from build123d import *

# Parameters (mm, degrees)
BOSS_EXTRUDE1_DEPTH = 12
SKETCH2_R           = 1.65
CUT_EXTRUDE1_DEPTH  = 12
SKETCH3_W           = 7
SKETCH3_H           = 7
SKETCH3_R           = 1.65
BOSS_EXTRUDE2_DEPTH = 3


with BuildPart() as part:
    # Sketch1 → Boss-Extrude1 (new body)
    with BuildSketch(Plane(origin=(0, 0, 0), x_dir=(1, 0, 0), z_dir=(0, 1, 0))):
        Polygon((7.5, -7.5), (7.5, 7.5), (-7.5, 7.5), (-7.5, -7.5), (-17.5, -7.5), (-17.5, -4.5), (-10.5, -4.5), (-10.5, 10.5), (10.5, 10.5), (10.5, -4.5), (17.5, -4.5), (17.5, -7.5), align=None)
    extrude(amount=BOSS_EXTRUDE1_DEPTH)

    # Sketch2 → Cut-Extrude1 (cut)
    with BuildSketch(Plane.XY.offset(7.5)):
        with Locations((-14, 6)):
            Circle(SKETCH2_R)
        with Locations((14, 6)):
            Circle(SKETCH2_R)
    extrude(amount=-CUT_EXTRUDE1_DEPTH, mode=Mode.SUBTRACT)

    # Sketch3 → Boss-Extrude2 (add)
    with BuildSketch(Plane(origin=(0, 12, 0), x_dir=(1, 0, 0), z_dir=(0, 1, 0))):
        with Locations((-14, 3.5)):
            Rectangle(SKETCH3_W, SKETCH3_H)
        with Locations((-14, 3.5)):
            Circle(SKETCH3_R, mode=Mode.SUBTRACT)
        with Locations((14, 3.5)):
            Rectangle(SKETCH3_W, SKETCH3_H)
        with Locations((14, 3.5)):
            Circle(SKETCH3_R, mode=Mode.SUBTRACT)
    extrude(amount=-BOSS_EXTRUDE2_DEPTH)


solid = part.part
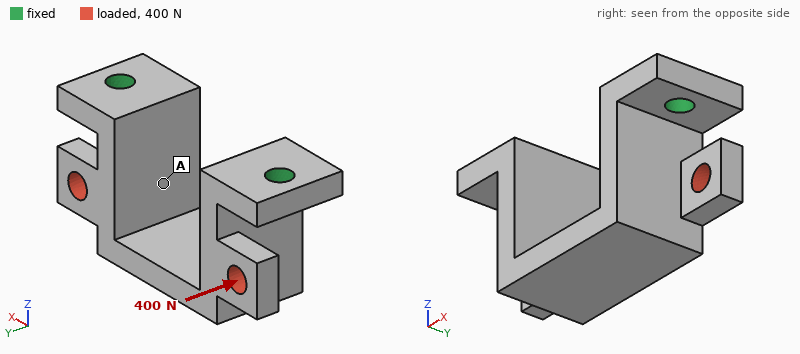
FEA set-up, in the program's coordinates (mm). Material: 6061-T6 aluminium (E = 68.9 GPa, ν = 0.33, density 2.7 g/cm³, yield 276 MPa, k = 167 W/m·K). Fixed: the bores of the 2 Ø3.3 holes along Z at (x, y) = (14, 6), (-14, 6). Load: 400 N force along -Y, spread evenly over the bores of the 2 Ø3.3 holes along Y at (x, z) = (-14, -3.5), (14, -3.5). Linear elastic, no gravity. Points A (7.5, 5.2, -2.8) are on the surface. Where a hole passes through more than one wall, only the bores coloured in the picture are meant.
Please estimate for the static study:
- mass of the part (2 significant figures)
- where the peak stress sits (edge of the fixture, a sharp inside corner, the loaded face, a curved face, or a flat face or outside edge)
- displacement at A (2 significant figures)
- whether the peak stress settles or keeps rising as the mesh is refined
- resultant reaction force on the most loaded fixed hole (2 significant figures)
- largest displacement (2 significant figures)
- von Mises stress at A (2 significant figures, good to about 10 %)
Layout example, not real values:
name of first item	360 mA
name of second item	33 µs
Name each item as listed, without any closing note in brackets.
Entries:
mass of the part	6.8 g
where the peak stress sits	edge of the fixture
displacement at A	26 µm
whether the peak stress settles or keeps rising as the mesh is refined	keeps rising
resultant reaction force on the most loaded fixed hole	200 N
largest displacement	69 µm
von Mises stress at A	17 MPa
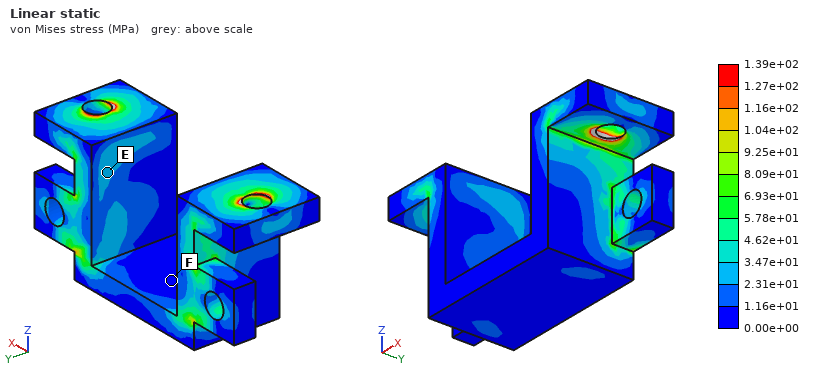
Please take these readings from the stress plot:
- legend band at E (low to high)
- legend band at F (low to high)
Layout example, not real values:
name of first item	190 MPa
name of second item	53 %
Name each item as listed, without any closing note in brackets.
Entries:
legend band at E	2.31e+01 to 3.47e+01 MPa
legend band at F	0.00e+00 to 1.16e+01 MPa
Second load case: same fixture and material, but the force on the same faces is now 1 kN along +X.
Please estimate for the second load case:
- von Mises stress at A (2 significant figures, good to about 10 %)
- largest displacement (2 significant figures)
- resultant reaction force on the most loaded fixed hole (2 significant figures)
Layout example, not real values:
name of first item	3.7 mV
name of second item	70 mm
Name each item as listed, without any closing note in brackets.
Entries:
von Mises stress at A	53 MPa
largest displacement	0.12 mm
resultant reaction force on the most loaded fixed hole	560 N
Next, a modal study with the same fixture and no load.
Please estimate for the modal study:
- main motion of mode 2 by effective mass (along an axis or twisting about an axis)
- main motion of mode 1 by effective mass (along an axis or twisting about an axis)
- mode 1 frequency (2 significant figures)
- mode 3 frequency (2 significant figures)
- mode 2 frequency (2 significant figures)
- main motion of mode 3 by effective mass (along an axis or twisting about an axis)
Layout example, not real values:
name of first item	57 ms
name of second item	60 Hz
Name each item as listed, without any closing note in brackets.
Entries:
main motion of mode 2 by effective mass	along X
main motion of mode 1 by effective mass	along Y
mode 1 frequency	6700 Hz
mode 3 frequency	10 kHz
mode 2 frequency	7800 Hz
main motion of mode 3 by effective mass	twisting about Z
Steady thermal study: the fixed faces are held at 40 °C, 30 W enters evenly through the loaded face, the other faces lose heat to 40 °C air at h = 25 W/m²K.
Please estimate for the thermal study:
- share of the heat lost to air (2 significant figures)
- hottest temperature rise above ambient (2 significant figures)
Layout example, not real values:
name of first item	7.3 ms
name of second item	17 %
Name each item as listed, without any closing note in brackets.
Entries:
share of the heat lost to air	4.4 %
hottest temperature rise above ambient	60 K
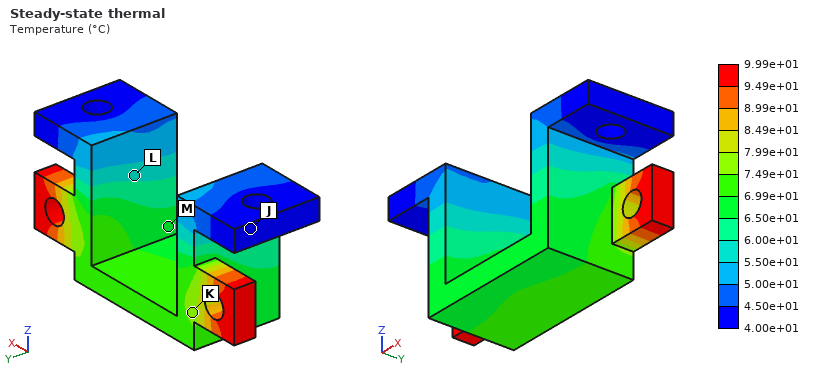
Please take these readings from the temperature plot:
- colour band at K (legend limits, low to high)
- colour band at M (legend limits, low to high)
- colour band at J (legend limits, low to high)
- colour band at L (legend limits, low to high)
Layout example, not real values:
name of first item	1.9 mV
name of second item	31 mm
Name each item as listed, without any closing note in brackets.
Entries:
colour band at K	7.49e+01 to 7.99e+01 °C
colour band at M	6.50e+01 to 6.99e+01 °C
colour band at J	4.00e+01 to 4.50e+01 °C
colour band at L	5.50e+01 to 6.00e+01 °C
